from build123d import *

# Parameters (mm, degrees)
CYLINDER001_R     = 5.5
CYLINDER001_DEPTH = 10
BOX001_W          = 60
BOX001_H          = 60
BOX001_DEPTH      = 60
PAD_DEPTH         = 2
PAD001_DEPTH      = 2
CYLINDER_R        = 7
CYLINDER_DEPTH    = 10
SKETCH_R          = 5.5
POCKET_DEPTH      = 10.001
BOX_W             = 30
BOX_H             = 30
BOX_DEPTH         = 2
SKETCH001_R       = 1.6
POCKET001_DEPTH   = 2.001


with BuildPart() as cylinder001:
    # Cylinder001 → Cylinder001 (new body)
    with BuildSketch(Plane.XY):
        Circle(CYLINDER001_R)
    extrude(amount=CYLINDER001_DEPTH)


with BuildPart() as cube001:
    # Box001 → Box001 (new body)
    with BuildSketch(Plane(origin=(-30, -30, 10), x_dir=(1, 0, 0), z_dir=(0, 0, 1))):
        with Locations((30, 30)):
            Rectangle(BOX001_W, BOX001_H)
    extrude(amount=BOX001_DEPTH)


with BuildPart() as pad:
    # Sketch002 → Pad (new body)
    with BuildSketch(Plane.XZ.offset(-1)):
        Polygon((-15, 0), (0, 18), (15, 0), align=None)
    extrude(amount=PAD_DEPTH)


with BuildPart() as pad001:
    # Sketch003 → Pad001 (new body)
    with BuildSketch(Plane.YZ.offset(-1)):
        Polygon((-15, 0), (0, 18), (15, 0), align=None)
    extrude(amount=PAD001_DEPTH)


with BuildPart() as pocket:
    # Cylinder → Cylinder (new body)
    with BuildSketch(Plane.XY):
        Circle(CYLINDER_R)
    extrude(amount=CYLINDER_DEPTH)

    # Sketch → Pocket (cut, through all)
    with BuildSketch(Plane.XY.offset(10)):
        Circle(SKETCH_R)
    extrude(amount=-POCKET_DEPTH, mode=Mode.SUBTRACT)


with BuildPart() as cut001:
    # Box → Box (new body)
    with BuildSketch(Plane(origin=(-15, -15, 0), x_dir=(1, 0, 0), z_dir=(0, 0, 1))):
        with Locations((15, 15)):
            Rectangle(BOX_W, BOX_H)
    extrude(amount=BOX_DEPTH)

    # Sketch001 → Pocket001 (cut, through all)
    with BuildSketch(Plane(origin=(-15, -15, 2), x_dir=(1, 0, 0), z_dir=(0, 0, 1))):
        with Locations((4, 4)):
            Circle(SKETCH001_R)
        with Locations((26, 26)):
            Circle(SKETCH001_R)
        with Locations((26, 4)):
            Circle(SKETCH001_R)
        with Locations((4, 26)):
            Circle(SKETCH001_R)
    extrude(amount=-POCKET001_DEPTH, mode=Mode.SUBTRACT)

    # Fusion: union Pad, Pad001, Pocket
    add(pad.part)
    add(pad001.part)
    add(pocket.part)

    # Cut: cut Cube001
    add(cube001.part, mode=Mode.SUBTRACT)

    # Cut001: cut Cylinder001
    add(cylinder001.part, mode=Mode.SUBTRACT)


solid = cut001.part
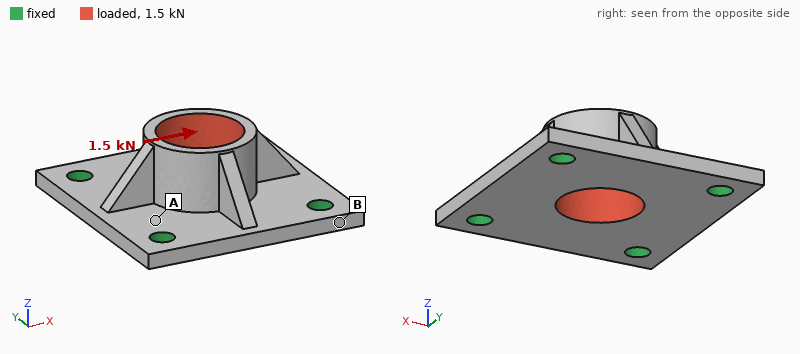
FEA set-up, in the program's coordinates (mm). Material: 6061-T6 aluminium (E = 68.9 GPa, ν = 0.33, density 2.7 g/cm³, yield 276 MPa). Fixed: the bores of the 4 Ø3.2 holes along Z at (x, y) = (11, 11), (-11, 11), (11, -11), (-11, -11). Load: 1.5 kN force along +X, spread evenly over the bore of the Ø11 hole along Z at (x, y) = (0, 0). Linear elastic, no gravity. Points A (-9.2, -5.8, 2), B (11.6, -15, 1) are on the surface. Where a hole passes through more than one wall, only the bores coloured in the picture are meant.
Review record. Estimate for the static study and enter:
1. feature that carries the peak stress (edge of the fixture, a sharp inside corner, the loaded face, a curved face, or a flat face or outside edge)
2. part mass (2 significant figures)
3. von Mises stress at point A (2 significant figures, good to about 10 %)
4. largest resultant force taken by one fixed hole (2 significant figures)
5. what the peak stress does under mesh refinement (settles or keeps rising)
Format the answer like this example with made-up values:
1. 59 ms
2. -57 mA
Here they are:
1. edge of the fixture
2. 6.0 g
3. 41 MPa
4. 430 N
5. keeps rising
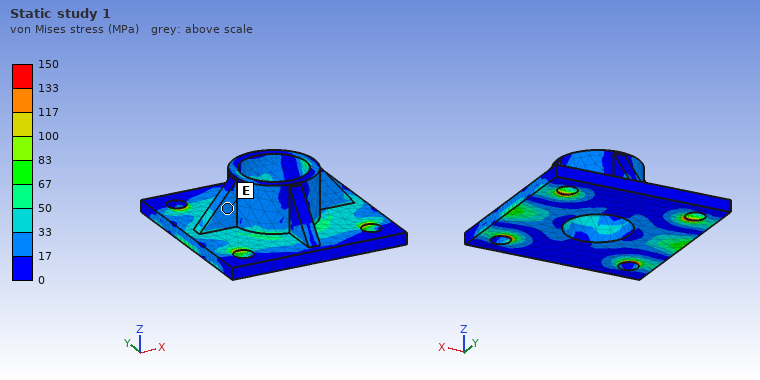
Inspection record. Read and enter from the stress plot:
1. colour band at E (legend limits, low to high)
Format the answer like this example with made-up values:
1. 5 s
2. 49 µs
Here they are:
1. 17 to 33 MPa
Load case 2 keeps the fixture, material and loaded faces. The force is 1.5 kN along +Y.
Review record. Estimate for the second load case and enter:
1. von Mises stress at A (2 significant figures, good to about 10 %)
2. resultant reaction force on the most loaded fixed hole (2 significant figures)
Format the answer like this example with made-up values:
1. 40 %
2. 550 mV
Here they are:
1. 42 MPa
2. 430 N
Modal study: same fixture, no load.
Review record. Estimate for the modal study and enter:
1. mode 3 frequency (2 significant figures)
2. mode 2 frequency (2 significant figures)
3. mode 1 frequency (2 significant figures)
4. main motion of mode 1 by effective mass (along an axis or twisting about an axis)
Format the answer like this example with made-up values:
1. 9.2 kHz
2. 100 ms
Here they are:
1. 20 kHz
2. 20 kHz
3. 17 kHz
4. along Z
